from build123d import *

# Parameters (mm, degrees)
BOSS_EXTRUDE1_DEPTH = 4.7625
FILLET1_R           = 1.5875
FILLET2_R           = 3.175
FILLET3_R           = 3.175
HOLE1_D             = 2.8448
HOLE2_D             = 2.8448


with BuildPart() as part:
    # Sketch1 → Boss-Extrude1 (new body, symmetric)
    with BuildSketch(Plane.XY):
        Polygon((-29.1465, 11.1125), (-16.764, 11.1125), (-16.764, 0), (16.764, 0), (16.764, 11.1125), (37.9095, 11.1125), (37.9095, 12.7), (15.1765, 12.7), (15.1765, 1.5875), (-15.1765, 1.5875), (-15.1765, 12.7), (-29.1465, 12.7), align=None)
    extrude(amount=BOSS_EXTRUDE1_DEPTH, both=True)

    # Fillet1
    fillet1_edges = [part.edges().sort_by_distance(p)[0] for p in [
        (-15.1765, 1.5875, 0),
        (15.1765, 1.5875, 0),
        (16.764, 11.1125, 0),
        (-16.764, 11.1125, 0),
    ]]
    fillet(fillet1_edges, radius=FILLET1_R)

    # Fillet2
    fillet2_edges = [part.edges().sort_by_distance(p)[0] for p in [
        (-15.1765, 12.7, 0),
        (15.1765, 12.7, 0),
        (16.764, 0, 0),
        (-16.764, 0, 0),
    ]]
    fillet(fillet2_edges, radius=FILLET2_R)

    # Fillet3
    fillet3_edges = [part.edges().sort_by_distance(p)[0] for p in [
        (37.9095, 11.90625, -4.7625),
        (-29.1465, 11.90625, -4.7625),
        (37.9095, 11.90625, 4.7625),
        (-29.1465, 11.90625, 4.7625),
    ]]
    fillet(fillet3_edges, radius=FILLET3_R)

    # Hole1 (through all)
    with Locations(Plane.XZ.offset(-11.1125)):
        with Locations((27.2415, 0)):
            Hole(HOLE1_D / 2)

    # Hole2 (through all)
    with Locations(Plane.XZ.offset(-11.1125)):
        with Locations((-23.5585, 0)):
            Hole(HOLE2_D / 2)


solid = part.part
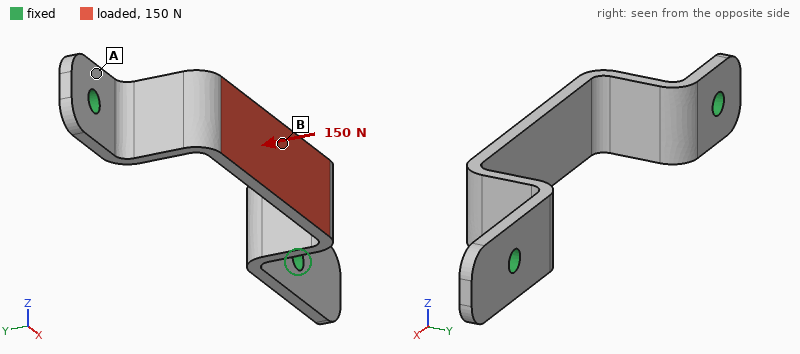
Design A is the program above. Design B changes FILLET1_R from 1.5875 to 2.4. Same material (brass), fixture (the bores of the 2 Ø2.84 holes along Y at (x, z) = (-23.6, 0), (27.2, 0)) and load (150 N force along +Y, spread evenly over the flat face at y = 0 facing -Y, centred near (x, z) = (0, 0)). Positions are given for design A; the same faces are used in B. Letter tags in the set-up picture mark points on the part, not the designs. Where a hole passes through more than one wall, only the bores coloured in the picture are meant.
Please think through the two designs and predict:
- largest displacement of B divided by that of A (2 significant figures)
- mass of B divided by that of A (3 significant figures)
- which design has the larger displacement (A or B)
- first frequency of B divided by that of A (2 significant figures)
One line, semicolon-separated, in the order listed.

0.82; 1.02; A; 1.0
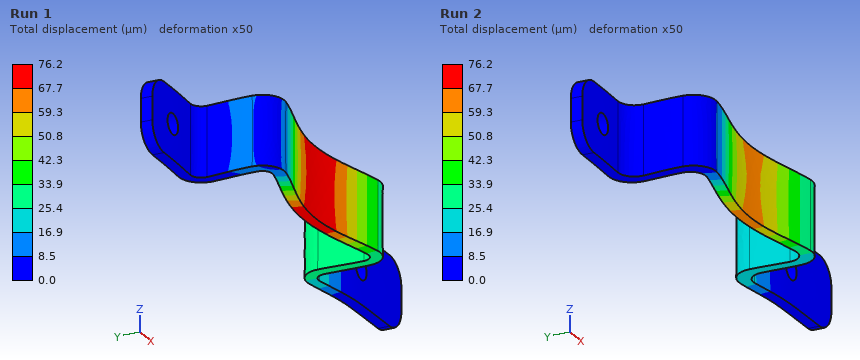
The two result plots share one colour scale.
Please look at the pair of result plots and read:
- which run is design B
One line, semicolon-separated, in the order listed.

Run 2
